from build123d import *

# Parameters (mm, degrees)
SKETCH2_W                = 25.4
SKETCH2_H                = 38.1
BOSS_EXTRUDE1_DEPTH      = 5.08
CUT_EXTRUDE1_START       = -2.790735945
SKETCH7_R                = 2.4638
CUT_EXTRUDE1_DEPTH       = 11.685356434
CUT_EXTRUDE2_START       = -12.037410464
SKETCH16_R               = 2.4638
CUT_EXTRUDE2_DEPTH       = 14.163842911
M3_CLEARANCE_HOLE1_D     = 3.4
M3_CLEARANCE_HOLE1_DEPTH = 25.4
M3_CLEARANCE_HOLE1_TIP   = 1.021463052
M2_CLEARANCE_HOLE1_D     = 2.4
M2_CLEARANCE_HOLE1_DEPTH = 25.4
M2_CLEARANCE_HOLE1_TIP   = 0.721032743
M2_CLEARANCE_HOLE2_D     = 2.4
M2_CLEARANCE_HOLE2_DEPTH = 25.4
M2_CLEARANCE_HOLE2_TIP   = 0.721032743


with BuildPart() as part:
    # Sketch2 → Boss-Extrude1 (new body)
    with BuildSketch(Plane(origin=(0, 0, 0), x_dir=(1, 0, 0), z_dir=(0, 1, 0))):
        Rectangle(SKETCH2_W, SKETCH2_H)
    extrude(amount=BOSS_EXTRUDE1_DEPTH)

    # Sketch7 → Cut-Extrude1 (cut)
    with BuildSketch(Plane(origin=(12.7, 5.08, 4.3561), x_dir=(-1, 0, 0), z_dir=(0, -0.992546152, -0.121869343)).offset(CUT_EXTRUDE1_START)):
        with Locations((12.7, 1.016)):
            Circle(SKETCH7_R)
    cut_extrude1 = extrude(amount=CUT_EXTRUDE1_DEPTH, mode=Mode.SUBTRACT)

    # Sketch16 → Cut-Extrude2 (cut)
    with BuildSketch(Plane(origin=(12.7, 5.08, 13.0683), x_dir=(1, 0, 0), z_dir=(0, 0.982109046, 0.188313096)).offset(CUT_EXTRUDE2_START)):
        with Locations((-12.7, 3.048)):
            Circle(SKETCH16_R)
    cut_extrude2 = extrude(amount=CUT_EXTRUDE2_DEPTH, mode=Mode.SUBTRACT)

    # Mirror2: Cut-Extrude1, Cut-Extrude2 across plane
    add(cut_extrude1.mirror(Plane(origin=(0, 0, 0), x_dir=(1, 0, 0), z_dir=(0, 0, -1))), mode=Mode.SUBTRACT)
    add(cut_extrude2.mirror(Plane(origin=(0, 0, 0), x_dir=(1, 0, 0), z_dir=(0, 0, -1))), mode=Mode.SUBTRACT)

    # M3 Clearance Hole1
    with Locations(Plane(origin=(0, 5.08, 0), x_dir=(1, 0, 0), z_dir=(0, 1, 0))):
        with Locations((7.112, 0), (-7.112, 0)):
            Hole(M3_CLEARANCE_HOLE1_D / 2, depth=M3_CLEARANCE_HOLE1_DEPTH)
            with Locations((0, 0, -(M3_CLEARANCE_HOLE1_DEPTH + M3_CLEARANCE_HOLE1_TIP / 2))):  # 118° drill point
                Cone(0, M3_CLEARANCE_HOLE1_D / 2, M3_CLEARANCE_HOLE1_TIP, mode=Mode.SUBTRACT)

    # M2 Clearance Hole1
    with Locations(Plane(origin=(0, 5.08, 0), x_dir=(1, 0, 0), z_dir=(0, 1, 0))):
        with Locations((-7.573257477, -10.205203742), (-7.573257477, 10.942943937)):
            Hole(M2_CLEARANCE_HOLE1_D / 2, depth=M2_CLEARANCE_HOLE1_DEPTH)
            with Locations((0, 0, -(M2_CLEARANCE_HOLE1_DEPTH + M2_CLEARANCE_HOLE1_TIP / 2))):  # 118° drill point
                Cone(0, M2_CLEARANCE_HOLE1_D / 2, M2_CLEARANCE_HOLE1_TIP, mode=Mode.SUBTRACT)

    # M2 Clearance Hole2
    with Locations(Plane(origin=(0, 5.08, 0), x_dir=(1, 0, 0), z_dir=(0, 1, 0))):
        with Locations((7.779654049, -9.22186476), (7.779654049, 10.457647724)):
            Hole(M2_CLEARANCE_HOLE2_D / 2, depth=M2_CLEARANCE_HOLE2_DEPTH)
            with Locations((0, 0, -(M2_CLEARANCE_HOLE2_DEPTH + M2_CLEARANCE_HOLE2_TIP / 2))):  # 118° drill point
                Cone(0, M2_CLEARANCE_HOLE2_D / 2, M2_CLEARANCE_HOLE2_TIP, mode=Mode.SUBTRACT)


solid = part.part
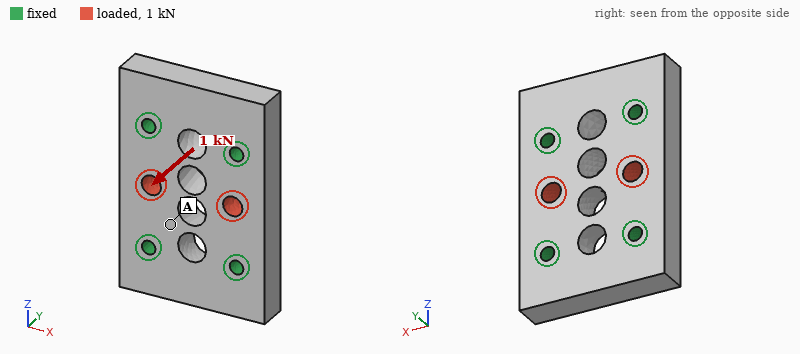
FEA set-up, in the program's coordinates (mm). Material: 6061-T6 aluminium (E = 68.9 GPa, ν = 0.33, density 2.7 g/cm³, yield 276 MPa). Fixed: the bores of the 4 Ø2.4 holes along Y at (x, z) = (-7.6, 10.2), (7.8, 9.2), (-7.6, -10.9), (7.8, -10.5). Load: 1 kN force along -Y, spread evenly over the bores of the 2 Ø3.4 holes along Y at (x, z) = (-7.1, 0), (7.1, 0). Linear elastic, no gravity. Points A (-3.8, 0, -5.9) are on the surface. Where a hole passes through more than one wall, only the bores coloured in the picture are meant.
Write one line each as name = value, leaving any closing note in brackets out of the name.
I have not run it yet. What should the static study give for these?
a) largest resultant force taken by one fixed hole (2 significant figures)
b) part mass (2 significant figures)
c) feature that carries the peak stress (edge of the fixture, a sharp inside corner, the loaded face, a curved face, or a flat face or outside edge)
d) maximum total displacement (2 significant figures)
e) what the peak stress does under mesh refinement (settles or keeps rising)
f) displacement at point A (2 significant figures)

largest resultant force taken by one fixed hole = 280 N
part mass = 12 g
feature that carries the peak stress = edge of the fixture
maximum total displacement = 6.3 µm
what the peak stress does under mesh refinement = keeps rising
displacement at point A = 3.1 µm
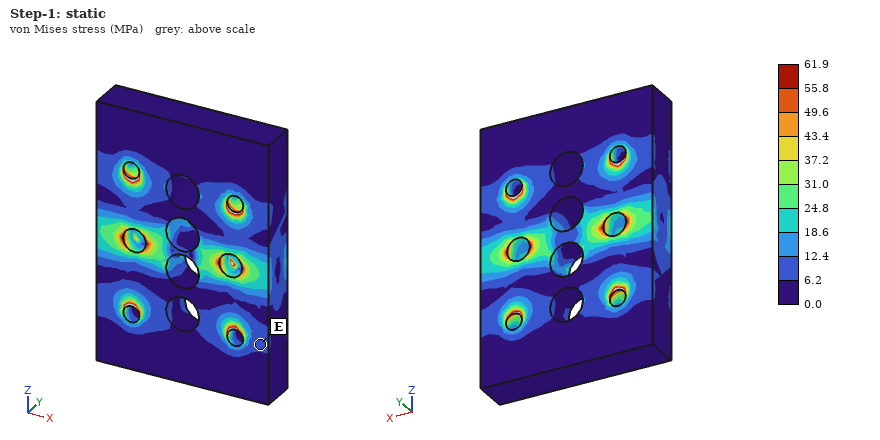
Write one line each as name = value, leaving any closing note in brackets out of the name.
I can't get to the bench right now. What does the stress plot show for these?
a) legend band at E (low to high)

legend band at E = 6.2 to 12.4 MPa
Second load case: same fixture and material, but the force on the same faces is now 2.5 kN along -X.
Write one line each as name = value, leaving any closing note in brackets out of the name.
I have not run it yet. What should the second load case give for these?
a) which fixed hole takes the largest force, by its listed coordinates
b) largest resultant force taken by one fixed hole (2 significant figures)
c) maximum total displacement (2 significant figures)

which fixed hole takes the largest force, by its listed coordinates = (7.8, 9.2)
largest resultant force taken by one fixed hole = 740 N
maximum total displacement = 7.1 µm
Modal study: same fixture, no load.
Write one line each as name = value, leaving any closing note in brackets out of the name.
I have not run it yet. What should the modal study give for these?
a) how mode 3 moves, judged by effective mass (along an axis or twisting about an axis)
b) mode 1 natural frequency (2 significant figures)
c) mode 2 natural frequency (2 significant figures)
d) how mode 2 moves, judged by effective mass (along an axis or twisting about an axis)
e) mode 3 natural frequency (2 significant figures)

how mode 3 moves, judged by effective mass = along Y
mode 1 natural frequency = 33 kHz
mode 2 natural frequency = 39 kHz
how mode 2 moves, judged by effective mass = twisting about X
mode 3 natural frequency = 44 kHz
